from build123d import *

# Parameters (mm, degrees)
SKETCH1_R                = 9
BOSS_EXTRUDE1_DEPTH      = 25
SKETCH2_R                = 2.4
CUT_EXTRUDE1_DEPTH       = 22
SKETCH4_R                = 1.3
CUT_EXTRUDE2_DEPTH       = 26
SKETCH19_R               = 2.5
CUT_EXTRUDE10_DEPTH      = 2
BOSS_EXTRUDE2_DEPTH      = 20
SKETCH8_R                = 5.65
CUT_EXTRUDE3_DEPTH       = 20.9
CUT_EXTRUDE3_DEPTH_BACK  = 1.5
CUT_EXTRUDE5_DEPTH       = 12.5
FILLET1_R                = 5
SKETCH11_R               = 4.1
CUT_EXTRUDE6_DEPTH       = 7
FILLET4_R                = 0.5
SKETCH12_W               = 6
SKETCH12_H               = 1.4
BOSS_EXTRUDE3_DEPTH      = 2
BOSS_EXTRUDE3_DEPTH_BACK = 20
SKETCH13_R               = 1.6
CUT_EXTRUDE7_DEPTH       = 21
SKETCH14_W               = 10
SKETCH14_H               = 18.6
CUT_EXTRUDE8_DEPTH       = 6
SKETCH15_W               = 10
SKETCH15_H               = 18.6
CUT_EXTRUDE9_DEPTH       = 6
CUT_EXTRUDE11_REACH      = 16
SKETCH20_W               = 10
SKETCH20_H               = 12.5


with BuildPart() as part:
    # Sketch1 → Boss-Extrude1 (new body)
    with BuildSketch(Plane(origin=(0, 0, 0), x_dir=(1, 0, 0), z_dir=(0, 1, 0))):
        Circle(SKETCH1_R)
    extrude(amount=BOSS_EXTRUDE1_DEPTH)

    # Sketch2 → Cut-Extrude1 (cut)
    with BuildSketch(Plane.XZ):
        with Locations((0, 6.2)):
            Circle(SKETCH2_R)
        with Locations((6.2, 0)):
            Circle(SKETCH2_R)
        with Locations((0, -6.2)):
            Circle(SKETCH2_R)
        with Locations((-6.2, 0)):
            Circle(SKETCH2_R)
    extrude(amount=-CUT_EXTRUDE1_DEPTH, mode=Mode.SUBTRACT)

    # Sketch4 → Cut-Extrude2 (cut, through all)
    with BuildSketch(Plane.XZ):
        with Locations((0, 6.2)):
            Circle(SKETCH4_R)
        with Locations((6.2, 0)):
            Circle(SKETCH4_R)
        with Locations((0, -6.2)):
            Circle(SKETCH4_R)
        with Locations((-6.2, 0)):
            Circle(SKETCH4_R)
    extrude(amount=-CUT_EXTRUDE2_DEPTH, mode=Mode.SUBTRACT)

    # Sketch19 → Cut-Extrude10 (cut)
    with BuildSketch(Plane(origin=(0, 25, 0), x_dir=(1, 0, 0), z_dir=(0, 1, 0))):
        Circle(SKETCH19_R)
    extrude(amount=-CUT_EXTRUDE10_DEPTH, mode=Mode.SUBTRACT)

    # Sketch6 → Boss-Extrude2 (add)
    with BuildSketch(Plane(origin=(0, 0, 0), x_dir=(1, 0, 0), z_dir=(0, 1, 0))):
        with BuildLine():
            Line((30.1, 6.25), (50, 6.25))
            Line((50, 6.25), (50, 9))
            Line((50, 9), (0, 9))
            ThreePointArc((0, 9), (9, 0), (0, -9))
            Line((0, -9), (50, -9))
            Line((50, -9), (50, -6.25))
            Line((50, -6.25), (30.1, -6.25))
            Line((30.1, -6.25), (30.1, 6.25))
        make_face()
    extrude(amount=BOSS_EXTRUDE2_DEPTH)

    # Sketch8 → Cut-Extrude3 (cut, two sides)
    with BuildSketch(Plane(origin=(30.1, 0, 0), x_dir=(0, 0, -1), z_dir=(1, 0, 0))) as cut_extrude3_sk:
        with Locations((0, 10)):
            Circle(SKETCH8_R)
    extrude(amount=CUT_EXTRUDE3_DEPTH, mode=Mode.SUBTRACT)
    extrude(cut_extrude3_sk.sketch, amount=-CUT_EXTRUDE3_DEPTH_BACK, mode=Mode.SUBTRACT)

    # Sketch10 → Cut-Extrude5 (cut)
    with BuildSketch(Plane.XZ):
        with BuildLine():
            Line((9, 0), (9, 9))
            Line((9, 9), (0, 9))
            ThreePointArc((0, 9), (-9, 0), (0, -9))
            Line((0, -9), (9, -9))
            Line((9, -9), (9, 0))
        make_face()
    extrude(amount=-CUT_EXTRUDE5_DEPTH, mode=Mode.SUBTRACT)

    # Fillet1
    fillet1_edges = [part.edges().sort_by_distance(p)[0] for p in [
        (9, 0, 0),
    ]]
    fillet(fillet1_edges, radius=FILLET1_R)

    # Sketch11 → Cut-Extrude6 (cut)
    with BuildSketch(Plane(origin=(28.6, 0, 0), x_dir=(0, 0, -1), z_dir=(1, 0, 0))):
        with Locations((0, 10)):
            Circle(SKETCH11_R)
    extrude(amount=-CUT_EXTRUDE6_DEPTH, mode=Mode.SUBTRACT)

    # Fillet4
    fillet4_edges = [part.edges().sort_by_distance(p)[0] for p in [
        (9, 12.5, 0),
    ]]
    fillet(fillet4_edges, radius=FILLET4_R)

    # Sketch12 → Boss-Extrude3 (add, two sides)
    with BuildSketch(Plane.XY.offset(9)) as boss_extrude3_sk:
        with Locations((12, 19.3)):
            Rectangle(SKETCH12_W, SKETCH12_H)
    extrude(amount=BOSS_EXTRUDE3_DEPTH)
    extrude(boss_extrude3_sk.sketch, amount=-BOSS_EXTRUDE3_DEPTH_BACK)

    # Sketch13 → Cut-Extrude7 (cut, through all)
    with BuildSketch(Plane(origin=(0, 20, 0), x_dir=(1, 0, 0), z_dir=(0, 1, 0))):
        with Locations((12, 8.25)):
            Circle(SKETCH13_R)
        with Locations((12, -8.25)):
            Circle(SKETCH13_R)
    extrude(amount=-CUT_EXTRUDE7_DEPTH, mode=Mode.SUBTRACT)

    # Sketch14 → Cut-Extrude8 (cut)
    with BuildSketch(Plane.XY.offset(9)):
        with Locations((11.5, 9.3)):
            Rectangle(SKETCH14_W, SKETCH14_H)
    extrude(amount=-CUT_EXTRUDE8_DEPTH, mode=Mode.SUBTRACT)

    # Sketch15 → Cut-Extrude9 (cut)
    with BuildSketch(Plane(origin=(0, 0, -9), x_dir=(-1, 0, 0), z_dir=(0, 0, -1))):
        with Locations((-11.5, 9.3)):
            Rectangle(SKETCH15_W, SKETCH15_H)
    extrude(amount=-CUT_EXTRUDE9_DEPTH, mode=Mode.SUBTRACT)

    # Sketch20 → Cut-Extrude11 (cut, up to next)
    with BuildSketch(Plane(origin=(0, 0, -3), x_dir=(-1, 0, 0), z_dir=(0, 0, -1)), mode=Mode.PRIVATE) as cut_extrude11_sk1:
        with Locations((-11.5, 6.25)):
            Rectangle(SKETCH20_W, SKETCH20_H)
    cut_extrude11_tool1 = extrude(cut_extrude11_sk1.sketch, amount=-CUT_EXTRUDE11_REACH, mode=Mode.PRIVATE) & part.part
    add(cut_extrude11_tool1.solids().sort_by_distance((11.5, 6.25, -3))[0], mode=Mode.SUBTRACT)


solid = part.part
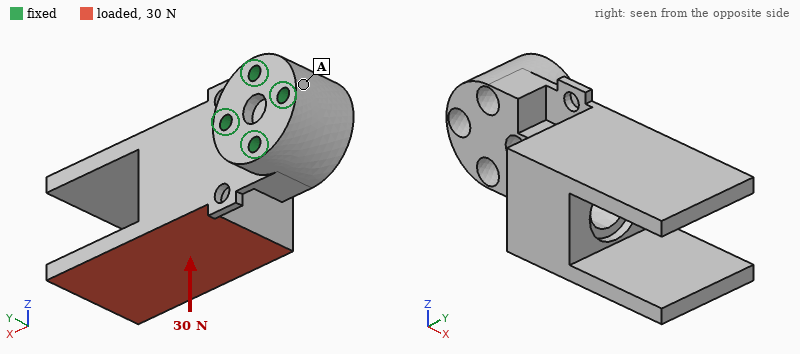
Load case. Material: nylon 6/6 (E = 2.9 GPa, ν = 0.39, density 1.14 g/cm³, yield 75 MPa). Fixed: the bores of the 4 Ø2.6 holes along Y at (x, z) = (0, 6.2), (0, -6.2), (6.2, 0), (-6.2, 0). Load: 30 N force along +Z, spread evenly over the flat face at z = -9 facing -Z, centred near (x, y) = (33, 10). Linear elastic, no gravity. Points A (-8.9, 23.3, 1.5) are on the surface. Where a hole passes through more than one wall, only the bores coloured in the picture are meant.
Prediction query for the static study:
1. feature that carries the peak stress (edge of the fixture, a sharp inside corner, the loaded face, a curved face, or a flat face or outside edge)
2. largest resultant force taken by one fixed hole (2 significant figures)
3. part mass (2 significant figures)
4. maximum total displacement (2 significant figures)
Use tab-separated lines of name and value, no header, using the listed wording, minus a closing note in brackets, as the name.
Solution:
feature that carries the peak stress	a curved face
largest resultant force taken by one fixed hole	55 N
part mass	11 g
maximum total displacement	0.63 mm
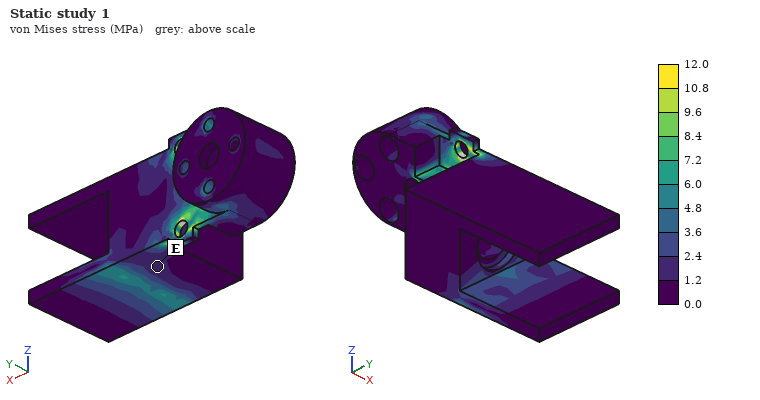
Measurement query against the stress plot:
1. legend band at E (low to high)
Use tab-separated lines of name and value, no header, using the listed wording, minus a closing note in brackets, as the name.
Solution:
legend band at E	1.2 to 2.4 MPa
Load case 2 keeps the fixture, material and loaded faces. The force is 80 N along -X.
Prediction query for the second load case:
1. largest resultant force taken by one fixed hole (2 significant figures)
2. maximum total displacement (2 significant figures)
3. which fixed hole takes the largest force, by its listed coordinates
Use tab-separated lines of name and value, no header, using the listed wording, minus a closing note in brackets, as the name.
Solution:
largest resultant force taken by one fixed hole	85 N
maximum total displacement	0.80 mm
which fixed hole takes the largest force, by its listed coordinates	(6.2, 0)
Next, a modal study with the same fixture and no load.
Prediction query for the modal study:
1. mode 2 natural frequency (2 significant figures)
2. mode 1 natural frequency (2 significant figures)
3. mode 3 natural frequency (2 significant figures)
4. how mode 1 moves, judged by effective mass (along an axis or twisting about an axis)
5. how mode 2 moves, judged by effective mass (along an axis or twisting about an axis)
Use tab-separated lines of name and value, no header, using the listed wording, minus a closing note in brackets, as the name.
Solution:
mode 2 natural frequency	670 Hz
mode 1 natural frequency	520 Hz
mode 3 natural frequency	1100 Hz
how mode 1 moves, judged by effective mass	along Y
how mode 2 moves, judged by effective mass	along Z
